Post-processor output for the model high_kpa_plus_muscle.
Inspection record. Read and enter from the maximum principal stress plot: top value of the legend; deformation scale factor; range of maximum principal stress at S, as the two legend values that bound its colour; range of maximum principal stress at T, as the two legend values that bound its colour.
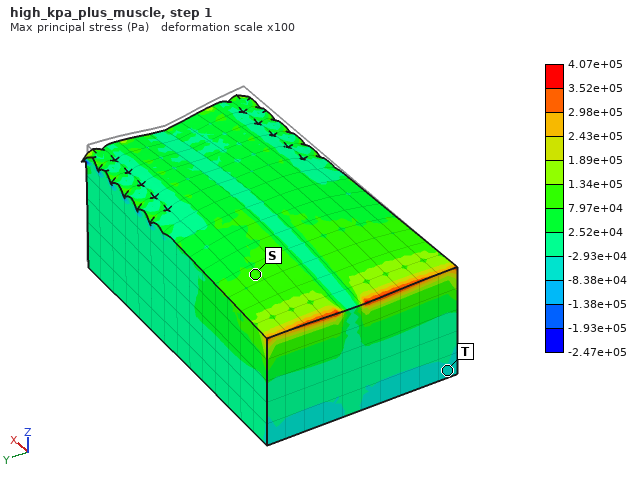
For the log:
4.07e+05 Pa
100
7.97e+04 to 1.34e+05 Pa
-8.38e+04 to -2.93e+04 Pa
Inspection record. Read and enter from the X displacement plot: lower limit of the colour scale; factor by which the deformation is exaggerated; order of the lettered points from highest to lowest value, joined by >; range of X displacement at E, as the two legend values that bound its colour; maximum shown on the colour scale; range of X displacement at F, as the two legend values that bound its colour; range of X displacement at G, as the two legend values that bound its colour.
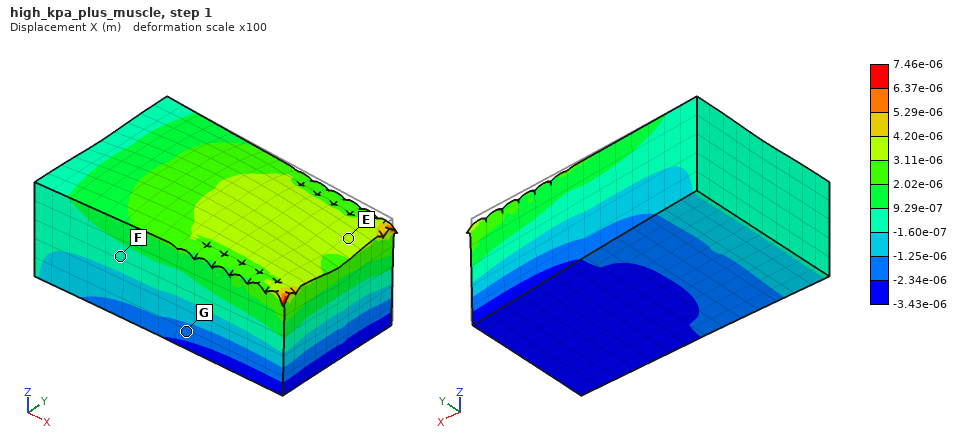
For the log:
-3.43e-06 m
100
E > F > G
3.11e-06 to 4.20e-06 m
7.46e-06 m
-1.60e-07 to 9.29e-07 m
-2.34e-06 to -1.25e-06 m
